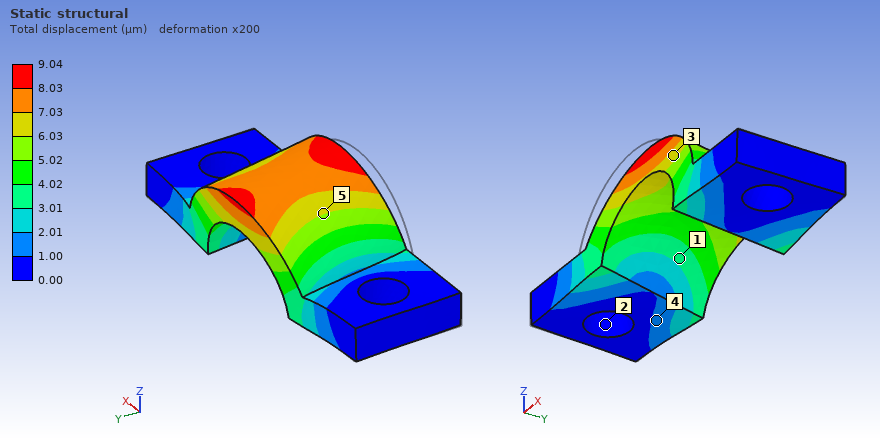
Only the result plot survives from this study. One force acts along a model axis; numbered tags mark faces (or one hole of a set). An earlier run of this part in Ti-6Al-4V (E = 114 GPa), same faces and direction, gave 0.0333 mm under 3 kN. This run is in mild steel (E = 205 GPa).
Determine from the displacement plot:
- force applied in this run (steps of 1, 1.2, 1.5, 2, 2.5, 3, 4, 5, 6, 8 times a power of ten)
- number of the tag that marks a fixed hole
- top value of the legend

1.5 kN
2
9.04 µm
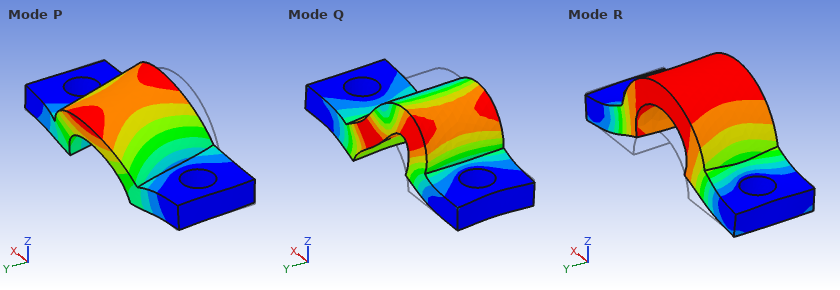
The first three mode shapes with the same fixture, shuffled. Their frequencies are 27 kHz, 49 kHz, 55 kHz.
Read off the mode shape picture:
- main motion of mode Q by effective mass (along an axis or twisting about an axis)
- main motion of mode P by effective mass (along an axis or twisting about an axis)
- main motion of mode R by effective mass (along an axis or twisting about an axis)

along X
along Y
along Z
